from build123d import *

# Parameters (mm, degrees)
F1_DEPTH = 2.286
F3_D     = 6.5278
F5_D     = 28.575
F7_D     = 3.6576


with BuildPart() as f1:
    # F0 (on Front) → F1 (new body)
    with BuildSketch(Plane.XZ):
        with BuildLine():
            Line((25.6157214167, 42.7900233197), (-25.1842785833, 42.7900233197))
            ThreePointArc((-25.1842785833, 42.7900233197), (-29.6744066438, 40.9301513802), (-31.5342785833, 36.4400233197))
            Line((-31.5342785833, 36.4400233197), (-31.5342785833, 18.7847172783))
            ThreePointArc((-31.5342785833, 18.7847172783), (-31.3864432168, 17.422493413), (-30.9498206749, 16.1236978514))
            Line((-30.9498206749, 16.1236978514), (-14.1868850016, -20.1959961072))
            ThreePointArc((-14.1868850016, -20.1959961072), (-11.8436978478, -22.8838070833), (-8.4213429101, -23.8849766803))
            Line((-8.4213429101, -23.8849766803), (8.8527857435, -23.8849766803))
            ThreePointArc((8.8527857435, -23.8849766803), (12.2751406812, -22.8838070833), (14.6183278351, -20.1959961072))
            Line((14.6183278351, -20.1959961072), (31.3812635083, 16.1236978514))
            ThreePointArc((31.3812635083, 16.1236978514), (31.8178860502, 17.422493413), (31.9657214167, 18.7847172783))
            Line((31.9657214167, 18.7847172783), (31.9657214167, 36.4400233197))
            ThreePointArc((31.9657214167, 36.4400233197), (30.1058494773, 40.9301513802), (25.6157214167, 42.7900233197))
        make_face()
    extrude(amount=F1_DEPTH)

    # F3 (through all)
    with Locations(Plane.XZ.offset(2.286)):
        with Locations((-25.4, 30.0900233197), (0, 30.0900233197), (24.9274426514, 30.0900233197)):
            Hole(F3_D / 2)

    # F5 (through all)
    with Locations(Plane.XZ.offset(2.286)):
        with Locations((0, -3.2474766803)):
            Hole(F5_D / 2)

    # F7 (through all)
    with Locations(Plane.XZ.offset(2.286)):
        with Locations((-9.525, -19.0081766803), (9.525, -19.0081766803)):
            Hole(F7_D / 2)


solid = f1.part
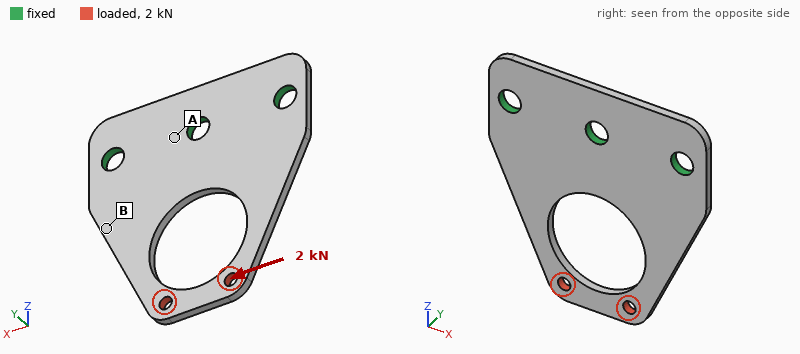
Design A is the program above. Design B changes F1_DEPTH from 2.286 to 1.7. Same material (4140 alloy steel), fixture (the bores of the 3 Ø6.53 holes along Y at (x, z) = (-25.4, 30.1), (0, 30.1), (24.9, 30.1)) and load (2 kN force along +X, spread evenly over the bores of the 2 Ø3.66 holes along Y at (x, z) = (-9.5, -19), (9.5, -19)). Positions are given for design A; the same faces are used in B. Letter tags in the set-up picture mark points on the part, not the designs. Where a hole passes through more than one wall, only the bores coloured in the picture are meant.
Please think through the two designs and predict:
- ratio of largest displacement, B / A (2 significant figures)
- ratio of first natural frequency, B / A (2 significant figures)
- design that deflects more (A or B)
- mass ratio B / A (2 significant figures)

1.3
0.75
B
0.74
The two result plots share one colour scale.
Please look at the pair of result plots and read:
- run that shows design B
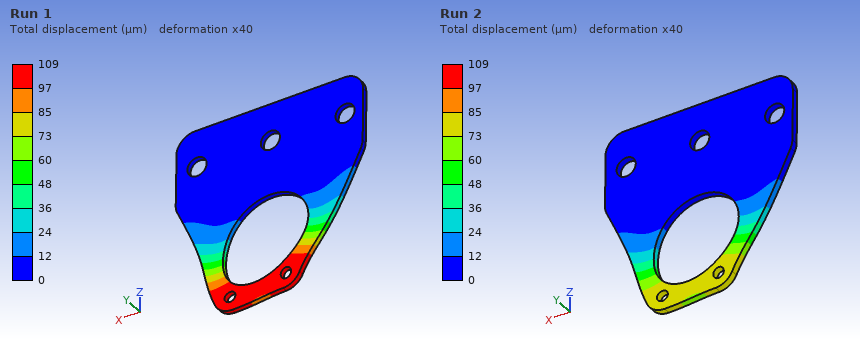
Run 1
